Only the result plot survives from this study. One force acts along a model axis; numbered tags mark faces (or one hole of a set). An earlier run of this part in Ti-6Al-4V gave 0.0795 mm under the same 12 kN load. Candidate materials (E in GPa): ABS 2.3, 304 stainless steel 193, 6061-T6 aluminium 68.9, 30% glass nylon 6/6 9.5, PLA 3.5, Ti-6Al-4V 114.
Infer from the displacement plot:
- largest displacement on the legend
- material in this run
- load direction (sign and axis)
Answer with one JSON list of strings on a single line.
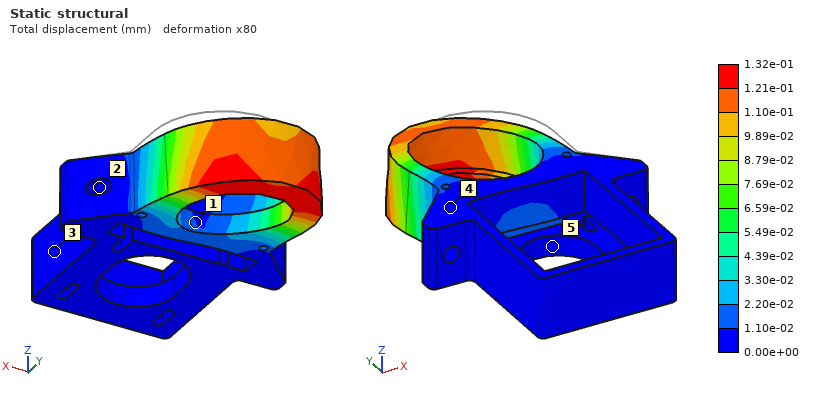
["1.32e-01 mm", "6061-T6 aluminium", "-X"]
